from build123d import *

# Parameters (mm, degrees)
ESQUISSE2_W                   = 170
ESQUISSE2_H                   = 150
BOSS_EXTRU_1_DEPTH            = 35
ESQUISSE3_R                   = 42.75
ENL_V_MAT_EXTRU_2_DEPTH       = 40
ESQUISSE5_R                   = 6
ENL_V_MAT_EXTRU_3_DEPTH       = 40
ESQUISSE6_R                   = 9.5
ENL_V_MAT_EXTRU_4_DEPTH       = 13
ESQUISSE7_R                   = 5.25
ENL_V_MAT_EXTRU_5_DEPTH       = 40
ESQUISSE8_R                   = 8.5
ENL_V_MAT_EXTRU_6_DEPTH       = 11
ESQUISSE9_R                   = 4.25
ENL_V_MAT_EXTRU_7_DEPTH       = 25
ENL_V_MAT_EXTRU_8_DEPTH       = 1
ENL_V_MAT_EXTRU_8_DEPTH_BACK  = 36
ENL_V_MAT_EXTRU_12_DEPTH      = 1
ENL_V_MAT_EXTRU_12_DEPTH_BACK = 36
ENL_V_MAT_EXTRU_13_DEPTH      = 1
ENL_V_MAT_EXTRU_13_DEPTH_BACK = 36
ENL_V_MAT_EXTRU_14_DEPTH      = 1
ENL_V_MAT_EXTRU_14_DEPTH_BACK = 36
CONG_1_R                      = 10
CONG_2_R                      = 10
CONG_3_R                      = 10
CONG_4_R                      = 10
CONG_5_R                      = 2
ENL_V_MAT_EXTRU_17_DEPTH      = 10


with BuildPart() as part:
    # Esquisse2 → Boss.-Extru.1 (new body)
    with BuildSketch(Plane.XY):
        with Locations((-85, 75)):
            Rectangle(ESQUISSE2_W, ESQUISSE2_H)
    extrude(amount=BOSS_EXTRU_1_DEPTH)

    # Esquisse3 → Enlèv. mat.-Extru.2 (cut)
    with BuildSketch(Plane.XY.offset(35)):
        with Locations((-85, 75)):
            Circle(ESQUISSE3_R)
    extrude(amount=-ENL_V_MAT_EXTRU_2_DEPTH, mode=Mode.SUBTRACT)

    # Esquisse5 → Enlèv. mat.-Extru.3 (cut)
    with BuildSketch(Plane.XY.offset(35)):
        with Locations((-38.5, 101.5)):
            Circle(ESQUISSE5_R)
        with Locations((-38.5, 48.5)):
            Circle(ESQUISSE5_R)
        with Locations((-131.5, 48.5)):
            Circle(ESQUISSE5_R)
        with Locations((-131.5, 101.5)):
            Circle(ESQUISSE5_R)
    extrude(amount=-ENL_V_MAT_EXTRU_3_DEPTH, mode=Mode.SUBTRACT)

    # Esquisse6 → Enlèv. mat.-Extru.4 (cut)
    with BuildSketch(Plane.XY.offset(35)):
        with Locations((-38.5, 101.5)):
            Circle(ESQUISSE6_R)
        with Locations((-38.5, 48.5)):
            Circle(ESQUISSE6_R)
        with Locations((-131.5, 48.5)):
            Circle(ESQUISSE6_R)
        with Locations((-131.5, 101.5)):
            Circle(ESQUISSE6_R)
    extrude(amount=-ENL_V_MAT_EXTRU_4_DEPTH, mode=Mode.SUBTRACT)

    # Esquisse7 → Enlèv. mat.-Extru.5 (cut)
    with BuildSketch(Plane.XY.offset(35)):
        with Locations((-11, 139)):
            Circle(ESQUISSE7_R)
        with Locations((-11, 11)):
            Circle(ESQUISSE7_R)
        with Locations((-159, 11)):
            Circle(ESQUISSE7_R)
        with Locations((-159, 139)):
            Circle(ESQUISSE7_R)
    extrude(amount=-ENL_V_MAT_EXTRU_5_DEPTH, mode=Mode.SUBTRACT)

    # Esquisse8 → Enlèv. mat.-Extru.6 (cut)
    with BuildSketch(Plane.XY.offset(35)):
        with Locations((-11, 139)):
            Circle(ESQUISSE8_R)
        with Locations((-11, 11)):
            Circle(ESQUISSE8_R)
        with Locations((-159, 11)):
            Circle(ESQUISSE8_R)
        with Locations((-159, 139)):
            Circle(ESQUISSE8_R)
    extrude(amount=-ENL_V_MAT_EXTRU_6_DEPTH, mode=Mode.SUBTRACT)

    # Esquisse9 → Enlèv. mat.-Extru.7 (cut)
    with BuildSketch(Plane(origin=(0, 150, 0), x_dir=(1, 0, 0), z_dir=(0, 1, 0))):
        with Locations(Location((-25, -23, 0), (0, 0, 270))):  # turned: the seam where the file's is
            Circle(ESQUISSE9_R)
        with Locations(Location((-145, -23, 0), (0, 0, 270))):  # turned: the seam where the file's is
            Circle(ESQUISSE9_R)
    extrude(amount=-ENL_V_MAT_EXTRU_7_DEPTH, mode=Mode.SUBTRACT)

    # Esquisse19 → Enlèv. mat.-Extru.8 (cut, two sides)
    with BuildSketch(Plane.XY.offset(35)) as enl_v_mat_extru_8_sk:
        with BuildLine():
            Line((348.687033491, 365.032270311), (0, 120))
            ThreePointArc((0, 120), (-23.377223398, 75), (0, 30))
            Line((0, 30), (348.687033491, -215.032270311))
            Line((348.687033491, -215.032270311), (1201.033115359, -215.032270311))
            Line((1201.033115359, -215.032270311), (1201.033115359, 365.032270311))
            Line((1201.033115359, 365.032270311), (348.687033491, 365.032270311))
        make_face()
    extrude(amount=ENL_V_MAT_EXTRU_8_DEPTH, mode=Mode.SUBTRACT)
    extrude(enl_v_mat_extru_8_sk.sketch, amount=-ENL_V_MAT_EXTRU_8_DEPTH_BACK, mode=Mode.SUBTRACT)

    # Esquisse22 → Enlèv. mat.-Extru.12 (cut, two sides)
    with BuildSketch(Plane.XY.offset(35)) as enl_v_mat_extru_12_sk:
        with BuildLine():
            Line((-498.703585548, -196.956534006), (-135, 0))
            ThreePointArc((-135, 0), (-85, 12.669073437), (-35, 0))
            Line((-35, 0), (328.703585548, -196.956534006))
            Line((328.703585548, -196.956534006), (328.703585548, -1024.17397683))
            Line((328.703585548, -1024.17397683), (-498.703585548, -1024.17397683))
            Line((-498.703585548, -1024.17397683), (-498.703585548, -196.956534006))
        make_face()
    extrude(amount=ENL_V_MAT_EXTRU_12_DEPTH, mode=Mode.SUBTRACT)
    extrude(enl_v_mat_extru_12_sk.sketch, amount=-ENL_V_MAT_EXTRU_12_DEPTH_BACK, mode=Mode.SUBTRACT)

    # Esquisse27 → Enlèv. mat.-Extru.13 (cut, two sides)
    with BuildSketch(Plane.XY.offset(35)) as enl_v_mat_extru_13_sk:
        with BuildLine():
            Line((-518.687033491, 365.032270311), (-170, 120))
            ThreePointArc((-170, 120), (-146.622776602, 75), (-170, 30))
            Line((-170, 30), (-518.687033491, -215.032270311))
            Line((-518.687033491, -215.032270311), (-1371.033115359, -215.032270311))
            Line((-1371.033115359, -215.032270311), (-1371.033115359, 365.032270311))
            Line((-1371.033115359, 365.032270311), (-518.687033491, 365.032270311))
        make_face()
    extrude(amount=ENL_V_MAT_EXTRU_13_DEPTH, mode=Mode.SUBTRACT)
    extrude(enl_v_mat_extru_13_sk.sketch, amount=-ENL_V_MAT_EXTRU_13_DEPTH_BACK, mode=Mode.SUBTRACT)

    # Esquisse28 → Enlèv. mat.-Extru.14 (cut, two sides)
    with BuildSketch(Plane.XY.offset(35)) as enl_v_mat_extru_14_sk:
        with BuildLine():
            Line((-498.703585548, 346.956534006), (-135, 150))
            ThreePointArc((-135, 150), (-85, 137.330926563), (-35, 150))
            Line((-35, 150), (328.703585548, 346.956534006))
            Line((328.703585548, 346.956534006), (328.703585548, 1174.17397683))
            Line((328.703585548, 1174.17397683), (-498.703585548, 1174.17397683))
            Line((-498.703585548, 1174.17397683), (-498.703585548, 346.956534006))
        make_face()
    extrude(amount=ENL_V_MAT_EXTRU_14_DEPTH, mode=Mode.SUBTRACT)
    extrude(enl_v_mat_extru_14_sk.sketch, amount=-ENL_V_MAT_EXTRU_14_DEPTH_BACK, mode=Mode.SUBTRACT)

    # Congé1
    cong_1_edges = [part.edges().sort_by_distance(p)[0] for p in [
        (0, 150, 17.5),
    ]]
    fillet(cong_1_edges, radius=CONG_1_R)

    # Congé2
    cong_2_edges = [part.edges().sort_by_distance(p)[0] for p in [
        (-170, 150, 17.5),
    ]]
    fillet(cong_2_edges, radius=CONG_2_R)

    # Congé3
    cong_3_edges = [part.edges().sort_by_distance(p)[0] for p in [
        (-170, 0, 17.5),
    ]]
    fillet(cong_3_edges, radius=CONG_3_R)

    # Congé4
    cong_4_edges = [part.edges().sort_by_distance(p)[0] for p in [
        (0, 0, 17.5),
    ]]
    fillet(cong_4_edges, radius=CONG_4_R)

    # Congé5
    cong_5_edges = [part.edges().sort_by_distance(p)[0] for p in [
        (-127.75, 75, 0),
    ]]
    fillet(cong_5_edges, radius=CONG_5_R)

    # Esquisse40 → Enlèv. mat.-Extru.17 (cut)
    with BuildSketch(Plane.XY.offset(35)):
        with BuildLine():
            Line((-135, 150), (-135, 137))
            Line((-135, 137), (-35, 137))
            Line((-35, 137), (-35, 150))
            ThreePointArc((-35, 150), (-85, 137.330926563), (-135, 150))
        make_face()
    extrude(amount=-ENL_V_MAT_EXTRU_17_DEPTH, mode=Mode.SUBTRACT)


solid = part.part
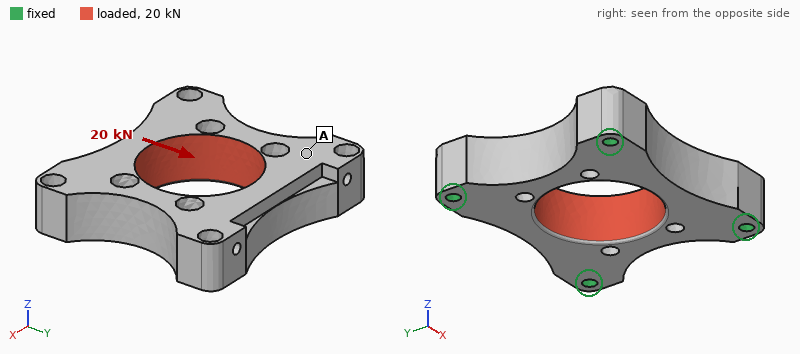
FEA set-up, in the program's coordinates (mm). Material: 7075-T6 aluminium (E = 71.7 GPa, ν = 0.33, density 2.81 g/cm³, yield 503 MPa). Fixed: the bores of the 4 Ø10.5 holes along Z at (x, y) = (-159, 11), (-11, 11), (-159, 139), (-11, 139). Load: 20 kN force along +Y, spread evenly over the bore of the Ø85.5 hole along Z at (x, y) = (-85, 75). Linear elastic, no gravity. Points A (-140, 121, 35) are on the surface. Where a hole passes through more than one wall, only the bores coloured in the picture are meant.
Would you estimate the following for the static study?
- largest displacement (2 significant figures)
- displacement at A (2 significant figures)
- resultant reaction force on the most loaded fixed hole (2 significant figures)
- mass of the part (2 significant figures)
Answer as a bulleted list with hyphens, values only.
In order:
- 18 µm
- 5.9 µm
- 6.2 kN
- 1.3 kg
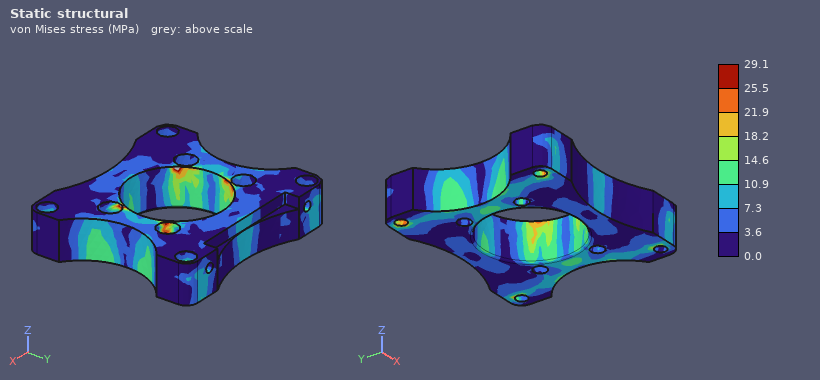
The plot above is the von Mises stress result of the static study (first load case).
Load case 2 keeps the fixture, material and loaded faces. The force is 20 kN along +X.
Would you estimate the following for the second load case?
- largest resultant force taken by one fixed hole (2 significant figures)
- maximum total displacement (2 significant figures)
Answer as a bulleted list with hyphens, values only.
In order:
- 5.9 kN
- 13 µm
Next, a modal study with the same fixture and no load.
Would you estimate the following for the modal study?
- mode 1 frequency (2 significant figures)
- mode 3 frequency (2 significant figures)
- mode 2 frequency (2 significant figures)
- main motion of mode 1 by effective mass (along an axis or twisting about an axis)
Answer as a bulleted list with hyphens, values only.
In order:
- 4500 Hz
- 6200 Hz
- 5900 Hz
- along Z
